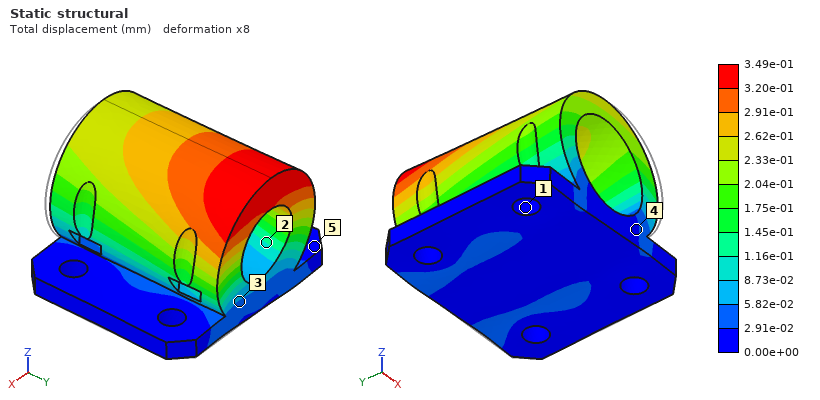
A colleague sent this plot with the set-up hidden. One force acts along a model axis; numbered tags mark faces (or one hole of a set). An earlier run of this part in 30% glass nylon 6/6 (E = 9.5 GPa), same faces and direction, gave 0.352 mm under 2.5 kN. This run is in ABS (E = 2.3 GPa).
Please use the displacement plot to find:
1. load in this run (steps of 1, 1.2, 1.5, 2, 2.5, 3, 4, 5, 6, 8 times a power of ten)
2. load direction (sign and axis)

600 N
-X
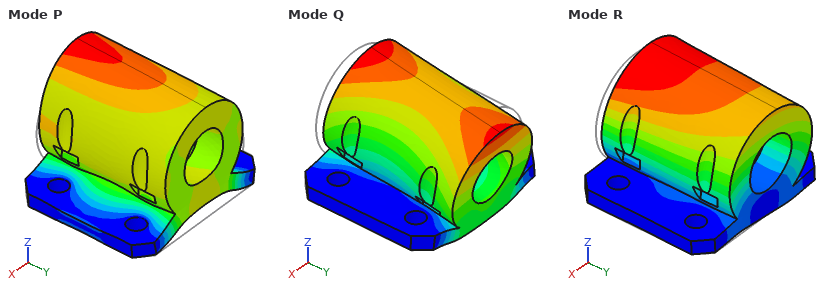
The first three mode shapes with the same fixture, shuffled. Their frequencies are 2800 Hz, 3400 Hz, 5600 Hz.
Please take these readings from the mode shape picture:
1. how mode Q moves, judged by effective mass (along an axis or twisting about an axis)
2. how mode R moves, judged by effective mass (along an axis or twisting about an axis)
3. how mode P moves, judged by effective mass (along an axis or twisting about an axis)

along Y
along X
along Z
